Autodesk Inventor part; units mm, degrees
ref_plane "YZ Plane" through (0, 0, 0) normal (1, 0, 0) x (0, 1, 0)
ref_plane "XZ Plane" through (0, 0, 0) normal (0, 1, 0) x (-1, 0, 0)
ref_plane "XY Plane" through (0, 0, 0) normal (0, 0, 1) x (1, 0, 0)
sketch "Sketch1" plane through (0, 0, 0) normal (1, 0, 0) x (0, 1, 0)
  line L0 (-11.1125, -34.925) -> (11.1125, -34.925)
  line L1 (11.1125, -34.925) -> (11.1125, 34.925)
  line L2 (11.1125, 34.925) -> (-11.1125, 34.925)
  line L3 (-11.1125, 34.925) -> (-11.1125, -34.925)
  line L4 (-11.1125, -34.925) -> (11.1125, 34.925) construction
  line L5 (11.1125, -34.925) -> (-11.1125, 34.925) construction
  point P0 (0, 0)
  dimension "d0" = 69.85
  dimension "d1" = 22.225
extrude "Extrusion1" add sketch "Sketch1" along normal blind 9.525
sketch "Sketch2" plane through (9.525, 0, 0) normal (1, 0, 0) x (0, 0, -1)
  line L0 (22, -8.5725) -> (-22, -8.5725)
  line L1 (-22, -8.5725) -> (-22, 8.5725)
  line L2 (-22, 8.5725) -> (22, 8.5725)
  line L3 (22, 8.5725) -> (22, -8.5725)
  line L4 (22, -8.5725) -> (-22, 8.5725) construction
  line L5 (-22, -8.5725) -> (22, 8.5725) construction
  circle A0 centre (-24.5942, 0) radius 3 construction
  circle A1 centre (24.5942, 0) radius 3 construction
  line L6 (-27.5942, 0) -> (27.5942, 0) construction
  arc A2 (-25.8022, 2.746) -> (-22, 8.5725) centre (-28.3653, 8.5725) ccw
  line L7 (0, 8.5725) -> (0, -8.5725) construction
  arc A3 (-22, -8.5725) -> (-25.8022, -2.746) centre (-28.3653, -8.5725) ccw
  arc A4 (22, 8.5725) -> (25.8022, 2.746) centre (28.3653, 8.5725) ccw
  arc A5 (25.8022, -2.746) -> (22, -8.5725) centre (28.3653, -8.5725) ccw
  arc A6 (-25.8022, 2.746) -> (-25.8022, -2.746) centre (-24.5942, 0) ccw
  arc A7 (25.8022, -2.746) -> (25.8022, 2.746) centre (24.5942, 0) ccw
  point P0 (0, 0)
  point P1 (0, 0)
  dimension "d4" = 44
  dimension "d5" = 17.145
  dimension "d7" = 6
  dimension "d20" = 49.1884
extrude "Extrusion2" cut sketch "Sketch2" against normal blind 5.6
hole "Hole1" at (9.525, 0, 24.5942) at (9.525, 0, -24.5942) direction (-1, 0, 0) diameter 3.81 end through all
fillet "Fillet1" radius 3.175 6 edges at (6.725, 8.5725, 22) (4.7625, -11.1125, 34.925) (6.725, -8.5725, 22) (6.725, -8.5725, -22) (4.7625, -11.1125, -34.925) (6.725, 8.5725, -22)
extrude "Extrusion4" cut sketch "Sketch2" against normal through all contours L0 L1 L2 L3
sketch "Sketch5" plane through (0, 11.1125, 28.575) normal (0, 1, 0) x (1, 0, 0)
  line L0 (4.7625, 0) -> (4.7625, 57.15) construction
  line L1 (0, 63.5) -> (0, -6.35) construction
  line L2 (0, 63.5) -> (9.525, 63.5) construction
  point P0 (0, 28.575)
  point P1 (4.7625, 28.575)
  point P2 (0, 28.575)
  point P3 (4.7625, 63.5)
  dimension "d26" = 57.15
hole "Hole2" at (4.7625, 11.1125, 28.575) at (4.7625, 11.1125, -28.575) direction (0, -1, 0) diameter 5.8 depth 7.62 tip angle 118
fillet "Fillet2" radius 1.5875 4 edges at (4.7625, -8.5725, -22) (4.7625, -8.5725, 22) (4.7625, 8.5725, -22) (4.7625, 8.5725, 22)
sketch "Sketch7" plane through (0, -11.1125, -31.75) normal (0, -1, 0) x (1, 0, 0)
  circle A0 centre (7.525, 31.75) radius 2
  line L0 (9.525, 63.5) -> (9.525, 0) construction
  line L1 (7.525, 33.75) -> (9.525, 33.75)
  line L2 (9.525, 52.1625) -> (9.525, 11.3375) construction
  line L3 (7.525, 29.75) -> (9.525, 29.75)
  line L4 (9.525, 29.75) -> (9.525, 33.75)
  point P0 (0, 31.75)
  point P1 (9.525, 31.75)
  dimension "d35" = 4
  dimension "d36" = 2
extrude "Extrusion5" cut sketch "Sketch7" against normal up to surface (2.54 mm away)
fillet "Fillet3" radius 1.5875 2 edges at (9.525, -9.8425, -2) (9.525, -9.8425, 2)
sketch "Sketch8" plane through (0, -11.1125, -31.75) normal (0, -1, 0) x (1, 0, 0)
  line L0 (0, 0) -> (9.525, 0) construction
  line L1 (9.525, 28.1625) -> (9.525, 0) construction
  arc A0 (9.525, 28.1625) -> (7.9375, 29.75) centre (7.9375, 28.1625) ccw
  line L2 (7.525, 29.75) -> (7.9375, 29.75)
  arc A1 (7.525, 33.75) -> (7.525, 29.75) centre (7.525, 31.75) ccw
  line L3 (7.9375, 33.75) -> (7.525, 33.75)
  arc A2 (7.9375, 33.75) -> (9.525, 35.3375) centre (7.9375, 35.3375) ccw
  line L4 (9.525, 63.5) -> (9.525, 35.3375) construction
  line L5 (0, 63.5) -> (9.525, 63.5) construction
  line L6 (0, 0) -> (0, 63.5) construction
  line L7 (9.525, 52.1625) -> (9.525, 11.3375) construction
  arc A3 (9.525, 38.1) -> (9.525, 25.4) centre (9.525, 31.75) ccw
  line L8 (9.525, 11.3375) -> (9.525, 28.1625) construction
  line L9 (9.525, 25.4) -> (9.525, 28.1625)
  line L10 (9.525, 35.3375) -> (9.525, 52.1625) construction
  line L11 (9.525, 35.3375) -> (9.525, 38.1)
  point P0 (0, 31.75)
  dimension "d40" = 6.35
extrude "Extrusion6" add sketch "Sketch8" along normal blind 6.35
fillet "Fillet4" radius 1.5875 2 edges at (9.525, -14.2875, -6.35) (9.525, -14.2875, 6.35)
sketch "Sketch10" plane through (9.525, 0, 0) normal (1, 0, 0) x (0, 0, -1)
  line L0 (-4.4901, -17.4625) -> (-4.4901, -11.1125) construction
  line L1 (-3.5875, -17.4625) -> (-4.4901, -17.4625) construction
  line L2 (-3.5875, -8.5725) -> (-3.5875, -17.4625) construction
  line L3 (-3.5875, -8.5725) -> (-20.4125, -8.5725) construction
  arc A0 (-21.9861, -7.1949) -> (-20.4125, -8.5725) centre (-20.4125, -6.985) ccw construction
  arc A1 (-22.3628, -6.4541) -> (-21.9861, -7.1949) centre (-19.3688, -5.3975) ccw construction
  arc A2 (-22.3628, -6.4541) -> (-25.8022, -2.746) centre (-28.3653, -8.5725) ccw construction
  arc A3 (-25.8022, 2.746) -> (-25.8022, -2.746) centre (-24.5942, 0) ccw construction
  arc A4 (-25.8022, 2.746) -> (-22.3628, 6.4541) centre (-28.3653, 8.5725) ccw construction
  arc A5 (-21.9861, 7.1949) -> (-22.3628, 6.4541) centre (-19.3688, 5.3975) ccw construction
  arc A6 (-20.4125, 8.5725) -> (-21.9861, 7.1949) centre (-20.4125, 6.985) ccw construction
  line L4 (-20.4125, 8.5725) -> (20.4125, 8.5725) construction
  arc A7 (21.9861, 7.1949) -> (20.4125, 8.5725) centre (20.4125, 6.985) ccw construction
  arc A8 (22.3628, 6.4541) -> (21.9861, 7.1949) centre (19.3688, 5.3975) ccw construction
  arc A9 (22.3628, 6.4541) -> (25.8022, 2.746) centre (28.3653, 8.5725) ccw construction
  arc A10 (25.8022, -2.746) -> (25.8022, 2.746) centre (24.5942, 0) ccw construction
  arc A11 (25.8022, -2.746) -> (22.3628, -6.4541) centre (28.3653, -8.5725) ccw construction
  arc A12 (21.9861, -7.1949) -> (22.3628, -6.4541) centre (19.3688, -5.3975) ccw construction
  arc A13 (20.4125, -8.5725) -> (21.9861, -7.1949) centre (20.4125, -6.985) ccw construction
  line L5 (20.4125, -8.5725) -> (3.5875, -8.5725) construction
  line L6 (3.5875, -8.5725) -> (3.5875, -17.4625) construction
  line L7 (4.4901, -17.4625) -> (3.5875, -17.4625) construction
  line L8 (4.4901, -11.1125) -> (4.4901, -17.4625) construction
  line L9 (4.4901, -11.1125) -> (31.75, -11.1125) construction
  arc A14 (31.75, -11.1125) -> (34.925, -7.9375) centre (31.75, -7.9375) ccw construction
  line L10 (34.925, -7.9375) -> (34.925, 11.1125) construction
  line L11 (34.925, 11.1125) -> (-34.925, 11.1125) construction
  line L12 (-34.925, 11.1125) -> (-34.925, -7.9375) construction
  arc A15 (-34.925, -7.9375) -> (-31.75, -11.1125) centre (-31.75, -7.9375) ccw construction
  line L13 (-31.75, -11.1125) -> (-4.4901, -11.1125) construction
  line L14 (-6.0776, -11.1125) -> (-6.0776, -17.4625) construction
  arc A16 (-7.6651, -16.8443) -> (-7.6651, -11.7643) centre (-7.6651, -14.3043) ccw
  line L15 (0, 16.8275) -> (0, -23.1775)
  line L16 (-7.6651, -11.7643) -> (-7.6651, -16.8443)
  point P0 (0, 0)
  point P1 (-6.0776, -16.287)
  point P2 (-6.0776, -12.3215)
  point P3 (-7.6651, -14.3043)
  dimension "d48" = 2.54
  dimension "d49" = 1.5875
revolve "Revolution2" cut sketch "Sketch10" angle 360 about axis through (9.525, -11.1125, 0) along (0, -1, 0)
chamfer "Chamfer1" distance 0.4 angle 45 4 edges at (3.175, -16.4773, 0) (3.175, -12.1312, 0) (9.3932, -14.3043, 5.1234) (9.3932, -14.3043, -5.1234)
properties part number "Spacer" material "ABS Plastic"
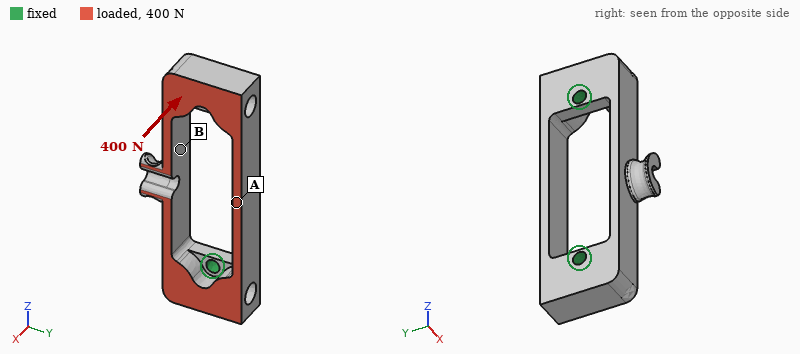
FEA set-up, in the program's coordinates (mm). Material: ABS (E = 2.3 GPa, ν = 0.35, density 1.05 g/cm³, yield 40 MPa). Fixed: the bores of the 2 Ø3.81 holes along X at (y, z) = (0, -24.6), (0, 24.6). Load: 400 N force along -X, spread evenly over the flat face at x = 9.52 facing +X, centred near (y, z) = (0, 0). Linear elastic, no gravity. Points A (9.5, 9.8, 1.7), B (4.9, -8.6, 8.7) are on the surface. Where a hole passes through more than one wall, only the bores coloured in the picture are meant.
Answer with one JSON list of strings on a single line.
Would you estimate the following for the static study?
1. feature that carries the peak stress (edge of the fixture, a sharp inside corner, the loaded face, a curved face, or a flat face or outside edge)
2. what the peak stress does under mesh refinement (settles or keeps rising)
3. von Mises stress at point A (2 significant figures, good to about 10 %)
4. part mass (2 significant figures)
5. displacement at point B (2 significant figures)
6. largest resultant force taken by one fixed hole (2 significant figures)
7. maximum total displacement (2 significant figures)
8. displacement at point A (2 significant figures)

["edge of the fixture", "keeps rising", "4.9 MPa", "7.1 g", "0.13 mm", "200 N", "0.24 mm", "0.16 mm"]
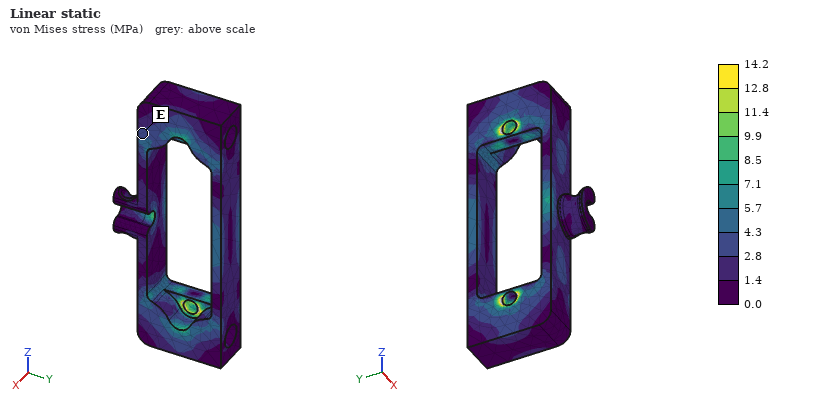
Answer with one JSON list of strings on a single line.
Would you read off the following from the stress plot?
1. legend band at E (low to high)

["2.8 to 4.3 MPa"]
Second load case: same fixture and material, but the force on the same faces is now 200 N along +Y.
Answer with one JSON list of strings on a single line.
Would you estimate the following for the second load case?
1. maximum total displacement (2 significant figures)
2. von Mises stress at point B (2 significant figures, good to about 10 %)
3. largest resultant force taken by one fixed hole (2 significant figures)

["0.48 mm", "4.0 MPa", "100 N"]
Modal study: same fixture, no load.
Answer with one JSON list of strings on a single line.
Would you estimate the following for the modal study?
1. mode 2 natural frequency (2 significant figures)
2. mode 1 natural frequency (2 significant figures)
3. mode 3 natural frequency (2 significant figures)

["1800 Hz", "1700 Hz", "2200 Hz"]
